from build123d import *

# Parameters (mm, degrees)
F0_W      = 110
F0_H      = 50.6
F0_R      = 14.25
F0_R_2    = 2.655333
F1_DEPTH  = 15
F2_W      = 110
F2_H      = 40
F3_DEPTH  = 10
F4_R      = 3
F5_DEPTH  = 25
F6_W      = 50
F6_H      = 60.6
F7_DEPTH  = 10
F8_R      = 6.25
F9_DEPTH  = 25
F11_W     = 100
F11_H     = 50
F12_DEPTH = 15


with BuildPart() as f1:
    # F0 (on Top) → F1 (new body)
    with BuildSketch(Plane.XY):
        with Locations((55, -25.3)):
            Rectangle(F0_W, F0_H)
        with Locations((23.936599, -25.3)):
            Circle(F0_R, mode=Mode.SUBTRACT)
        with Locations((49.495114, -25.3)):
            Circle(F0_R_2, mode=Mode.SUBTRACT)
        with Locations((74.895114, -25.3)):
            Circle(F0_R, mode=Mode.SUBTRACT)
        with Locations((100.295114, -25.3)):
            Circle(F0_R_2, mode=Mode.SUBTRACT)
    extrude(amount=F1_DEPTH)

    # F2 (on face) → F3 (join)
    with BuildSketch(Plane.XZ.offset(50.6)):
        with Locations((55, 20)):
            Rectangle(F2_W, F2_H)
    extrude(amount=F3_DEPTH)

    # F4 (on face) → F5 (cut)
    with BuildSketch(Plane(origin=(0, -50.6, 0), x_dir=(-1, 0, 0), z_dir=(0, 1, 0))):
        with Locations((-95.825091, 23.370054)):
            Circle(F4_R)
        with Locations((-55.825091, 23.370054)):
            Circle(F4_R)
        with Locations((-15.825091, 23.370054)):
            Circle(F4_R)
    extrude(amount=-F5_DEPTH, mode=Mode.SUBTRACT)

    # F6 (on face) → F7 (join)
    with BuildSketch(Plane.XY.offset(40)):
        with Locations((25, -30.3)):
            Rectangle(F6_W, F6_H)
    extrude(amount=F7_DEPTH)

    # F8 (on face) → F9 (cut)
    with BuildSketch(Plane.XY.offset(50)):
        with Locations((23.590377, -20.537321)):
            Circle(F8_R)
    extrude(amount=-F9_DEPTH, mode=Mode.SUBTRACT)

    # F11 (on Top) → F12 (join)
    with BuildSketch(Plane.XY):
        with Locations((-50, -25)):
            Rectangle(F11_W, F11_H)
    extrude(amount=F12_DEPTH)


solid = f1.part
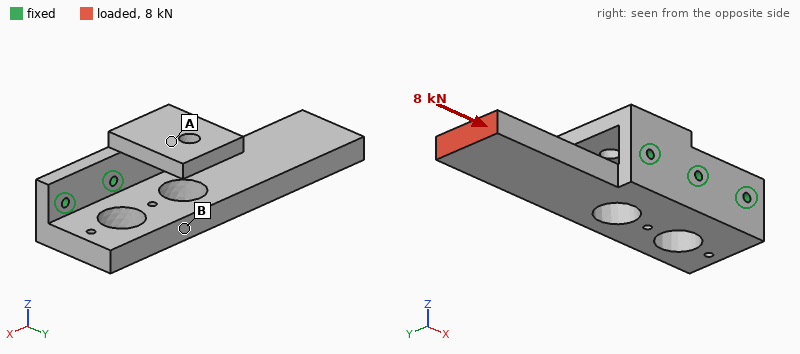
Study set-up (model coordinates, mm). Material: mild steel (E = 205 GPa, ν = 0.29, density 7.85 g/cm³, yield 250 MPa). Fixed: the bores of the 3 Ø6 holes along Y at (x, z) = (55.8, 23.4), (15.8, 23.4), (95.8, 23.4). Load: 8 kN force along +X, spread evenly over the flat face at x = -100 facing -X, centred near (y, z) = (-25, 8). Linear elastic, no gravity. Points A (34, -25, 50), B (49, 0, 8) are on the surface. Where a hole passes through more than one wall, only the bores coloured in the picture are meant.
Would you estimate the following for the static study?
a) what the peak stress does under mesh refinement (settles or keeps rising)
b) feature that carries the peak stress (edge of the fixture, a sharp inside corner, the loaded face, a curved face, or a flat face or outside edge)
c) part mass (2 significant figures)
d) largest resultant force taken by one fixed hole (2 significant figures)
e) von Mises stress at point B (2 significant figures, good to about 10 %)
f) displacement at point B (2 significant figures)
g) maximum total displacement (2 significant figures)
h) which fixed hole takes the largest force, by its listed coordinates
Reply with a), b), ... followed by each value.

a) keeps rising
b) edge of the fixture
c) 1.7 kg
d) 4.6 kN
e) 19 MPa
f) 16 µm
g) 54 µm
h) (15.8, 23.4)
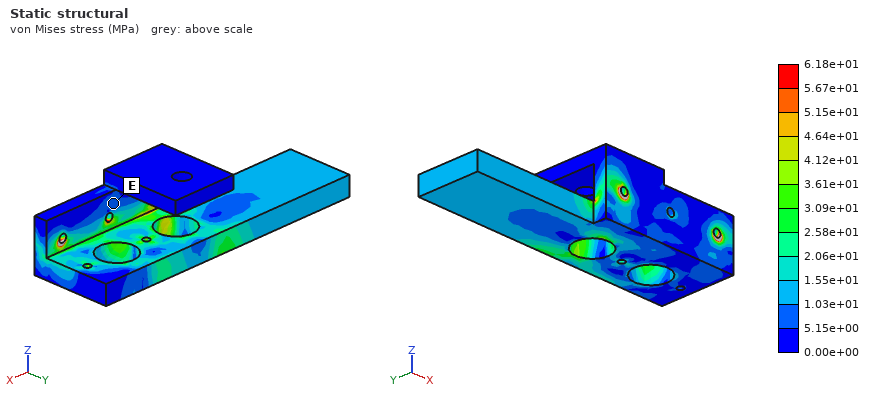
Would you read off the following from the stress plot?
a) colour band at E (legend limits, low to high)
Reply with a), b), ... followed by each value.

a) 5.15e+00 to 1.03e+01 MPa
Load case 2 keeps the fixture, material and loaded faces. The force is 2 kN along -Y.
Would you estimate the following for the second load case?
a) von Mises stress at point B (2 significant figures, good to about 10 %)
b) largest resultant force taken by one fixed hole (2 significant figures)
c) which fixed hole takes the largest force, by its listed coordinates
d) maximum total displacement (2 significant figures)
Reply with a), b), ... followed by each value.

a) 19 MPa
b) 4.8 kN
c) (15.8, 23.4)
d) 0.12 mm
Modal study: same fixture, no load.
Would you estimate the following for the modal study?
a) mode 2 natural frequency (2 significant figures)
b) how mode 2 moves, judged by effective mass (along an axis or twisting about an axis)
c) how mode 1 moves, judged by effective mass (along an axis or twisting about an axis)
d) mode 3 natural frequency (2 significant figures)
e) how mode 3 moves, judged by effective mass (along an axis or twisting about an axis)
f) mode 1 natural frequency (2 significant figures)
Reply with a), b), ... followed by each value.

a) 1400 Hz
b) along Y
c) along Z
d) 1700 Hz
e) along Z
f) 630 Hz
